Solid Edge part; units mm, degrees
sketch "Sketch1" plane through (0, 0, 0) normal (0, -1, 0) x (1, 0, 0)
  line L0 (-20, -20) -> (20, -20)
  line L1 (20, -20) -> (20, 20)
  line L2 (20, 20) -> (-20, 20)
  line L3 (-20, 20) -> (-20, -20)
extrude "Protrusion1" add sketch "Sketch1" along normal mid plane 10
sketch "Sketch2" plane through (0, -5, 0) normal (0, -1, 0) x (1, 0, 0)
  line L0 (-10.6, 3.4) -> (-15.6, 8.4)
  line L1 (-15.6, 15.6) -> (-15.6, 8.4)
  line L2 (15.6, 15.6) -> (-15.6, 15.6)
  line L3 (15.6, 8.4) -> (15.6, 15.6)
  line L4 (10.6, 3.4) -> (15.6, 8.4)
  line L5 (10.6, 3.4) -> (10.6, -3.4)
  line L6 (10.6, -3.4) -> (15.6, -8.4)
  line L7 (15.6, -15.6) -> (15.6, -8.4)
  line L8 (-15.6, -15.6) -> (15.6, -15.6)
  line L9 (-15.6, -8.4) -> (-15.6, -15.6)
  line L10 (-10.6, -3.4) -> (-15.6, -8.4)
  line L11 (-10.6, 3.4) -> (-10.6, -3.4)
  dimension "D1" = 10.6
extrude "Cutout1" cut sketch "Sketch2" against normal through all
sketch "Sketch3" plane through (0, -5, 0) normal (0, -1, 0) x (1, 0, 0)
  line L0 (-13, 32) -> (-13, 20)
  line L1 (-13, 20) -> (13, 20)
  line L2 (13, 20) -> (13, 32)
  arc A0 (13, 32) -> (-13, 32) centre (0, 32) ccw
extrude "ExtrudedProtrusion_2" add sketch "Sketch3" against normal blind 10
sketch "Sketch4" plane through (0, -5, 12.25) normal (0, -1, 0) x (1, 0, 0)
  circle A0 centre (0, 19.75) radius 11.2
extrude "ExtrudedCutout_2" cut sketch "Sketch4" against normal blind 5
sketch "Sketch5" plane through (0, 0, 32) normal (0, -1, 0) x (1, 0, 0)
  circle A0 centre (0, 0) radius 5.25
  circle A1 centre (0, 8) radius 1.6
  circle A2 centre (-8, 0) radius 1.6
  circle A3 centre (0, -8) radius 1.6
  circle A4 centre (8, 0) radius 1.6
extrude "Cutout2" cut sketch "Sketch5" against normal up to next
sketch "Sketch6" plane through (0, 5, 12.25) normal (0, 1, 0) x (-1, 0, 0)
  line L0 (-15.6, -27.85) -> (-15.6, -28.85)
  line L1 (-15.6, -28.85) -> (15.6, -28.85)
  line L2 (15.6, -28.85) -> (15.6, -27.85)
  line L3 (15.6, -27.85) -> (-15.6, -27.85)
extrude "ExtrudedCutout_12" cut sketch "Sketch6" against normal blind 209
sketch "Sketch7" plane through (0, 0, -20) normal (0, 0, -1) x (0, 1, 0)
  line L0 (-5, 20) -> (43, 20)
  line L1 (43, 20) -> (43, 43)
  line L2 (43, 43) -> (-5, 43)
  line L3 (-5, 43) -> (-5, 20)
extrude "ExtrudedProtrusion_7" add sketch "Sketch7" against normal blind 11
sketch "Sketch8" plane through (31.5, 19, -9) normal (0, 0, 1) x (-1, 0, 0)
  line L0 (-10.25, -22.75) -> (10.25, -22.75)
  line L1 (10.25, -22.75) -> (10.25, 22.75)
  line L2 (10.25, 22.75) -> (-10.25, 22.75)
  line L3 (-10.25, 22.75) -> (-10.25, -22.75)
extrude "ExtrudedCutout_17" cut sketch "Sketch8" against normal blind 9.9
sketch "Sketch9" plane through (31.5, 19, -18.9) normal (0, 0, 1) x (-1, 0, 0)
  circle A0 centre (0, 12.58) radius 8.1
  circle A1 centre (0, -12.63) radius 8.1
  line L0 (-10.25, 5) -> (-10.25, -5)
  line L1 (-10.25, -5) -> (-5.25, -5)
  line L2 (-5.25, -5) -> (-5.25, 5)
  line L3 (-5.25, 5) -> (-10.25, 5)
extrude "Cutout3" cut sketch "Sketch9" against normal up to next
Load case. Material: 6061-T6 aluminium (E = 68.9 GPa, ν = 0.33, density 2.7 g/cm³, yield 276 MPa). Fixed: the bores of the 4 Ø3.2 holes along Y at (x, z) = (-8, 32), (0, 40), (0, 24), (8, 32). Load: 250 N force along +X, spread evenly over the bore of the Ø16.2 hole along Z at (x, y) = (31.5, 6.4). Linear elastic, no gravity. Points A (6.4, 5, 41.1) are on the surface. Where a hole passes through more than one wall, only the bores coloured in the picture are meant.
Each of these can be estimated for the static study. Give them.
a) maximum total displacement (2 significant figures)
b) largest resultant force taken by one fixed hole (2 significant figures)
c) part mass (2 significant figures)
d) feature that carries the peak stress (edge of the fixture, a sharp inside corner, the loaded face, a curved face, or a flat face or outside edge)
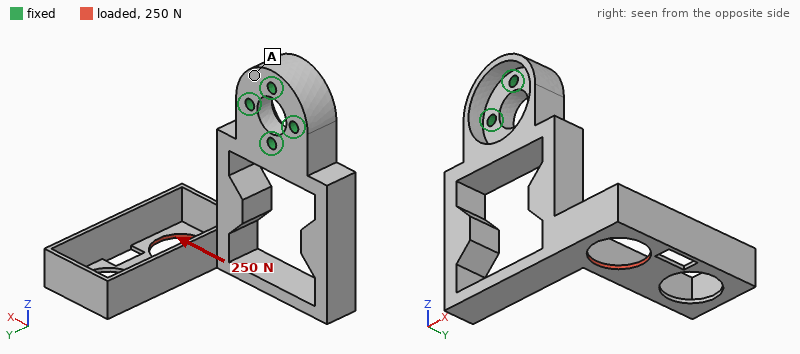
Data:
0.58 mm
500 N
34 g
the loaded face
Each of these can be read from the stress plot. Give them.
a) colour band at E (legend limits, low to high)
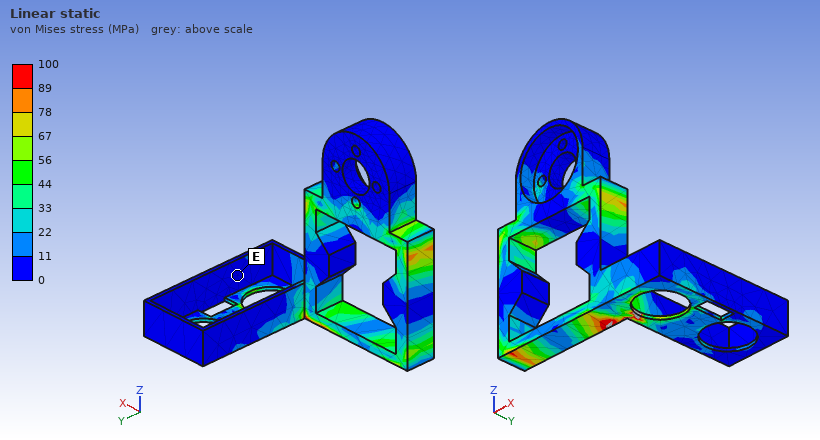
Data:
0 to 11 MPa
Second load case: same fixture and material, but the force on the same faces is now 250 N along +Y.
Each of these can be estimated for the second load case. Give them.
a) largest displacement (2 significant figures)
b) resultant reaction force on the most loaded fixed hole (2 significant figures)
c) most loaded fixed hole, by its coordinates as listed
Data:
1.2 mm
790 N
(0, 24)
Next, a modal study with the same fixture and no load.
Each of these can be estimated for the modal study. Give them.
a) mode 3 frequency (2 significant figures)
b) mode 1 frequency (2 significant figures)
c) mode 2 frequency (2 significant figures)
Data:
1300 Hz
830 Hz
980 Hz
